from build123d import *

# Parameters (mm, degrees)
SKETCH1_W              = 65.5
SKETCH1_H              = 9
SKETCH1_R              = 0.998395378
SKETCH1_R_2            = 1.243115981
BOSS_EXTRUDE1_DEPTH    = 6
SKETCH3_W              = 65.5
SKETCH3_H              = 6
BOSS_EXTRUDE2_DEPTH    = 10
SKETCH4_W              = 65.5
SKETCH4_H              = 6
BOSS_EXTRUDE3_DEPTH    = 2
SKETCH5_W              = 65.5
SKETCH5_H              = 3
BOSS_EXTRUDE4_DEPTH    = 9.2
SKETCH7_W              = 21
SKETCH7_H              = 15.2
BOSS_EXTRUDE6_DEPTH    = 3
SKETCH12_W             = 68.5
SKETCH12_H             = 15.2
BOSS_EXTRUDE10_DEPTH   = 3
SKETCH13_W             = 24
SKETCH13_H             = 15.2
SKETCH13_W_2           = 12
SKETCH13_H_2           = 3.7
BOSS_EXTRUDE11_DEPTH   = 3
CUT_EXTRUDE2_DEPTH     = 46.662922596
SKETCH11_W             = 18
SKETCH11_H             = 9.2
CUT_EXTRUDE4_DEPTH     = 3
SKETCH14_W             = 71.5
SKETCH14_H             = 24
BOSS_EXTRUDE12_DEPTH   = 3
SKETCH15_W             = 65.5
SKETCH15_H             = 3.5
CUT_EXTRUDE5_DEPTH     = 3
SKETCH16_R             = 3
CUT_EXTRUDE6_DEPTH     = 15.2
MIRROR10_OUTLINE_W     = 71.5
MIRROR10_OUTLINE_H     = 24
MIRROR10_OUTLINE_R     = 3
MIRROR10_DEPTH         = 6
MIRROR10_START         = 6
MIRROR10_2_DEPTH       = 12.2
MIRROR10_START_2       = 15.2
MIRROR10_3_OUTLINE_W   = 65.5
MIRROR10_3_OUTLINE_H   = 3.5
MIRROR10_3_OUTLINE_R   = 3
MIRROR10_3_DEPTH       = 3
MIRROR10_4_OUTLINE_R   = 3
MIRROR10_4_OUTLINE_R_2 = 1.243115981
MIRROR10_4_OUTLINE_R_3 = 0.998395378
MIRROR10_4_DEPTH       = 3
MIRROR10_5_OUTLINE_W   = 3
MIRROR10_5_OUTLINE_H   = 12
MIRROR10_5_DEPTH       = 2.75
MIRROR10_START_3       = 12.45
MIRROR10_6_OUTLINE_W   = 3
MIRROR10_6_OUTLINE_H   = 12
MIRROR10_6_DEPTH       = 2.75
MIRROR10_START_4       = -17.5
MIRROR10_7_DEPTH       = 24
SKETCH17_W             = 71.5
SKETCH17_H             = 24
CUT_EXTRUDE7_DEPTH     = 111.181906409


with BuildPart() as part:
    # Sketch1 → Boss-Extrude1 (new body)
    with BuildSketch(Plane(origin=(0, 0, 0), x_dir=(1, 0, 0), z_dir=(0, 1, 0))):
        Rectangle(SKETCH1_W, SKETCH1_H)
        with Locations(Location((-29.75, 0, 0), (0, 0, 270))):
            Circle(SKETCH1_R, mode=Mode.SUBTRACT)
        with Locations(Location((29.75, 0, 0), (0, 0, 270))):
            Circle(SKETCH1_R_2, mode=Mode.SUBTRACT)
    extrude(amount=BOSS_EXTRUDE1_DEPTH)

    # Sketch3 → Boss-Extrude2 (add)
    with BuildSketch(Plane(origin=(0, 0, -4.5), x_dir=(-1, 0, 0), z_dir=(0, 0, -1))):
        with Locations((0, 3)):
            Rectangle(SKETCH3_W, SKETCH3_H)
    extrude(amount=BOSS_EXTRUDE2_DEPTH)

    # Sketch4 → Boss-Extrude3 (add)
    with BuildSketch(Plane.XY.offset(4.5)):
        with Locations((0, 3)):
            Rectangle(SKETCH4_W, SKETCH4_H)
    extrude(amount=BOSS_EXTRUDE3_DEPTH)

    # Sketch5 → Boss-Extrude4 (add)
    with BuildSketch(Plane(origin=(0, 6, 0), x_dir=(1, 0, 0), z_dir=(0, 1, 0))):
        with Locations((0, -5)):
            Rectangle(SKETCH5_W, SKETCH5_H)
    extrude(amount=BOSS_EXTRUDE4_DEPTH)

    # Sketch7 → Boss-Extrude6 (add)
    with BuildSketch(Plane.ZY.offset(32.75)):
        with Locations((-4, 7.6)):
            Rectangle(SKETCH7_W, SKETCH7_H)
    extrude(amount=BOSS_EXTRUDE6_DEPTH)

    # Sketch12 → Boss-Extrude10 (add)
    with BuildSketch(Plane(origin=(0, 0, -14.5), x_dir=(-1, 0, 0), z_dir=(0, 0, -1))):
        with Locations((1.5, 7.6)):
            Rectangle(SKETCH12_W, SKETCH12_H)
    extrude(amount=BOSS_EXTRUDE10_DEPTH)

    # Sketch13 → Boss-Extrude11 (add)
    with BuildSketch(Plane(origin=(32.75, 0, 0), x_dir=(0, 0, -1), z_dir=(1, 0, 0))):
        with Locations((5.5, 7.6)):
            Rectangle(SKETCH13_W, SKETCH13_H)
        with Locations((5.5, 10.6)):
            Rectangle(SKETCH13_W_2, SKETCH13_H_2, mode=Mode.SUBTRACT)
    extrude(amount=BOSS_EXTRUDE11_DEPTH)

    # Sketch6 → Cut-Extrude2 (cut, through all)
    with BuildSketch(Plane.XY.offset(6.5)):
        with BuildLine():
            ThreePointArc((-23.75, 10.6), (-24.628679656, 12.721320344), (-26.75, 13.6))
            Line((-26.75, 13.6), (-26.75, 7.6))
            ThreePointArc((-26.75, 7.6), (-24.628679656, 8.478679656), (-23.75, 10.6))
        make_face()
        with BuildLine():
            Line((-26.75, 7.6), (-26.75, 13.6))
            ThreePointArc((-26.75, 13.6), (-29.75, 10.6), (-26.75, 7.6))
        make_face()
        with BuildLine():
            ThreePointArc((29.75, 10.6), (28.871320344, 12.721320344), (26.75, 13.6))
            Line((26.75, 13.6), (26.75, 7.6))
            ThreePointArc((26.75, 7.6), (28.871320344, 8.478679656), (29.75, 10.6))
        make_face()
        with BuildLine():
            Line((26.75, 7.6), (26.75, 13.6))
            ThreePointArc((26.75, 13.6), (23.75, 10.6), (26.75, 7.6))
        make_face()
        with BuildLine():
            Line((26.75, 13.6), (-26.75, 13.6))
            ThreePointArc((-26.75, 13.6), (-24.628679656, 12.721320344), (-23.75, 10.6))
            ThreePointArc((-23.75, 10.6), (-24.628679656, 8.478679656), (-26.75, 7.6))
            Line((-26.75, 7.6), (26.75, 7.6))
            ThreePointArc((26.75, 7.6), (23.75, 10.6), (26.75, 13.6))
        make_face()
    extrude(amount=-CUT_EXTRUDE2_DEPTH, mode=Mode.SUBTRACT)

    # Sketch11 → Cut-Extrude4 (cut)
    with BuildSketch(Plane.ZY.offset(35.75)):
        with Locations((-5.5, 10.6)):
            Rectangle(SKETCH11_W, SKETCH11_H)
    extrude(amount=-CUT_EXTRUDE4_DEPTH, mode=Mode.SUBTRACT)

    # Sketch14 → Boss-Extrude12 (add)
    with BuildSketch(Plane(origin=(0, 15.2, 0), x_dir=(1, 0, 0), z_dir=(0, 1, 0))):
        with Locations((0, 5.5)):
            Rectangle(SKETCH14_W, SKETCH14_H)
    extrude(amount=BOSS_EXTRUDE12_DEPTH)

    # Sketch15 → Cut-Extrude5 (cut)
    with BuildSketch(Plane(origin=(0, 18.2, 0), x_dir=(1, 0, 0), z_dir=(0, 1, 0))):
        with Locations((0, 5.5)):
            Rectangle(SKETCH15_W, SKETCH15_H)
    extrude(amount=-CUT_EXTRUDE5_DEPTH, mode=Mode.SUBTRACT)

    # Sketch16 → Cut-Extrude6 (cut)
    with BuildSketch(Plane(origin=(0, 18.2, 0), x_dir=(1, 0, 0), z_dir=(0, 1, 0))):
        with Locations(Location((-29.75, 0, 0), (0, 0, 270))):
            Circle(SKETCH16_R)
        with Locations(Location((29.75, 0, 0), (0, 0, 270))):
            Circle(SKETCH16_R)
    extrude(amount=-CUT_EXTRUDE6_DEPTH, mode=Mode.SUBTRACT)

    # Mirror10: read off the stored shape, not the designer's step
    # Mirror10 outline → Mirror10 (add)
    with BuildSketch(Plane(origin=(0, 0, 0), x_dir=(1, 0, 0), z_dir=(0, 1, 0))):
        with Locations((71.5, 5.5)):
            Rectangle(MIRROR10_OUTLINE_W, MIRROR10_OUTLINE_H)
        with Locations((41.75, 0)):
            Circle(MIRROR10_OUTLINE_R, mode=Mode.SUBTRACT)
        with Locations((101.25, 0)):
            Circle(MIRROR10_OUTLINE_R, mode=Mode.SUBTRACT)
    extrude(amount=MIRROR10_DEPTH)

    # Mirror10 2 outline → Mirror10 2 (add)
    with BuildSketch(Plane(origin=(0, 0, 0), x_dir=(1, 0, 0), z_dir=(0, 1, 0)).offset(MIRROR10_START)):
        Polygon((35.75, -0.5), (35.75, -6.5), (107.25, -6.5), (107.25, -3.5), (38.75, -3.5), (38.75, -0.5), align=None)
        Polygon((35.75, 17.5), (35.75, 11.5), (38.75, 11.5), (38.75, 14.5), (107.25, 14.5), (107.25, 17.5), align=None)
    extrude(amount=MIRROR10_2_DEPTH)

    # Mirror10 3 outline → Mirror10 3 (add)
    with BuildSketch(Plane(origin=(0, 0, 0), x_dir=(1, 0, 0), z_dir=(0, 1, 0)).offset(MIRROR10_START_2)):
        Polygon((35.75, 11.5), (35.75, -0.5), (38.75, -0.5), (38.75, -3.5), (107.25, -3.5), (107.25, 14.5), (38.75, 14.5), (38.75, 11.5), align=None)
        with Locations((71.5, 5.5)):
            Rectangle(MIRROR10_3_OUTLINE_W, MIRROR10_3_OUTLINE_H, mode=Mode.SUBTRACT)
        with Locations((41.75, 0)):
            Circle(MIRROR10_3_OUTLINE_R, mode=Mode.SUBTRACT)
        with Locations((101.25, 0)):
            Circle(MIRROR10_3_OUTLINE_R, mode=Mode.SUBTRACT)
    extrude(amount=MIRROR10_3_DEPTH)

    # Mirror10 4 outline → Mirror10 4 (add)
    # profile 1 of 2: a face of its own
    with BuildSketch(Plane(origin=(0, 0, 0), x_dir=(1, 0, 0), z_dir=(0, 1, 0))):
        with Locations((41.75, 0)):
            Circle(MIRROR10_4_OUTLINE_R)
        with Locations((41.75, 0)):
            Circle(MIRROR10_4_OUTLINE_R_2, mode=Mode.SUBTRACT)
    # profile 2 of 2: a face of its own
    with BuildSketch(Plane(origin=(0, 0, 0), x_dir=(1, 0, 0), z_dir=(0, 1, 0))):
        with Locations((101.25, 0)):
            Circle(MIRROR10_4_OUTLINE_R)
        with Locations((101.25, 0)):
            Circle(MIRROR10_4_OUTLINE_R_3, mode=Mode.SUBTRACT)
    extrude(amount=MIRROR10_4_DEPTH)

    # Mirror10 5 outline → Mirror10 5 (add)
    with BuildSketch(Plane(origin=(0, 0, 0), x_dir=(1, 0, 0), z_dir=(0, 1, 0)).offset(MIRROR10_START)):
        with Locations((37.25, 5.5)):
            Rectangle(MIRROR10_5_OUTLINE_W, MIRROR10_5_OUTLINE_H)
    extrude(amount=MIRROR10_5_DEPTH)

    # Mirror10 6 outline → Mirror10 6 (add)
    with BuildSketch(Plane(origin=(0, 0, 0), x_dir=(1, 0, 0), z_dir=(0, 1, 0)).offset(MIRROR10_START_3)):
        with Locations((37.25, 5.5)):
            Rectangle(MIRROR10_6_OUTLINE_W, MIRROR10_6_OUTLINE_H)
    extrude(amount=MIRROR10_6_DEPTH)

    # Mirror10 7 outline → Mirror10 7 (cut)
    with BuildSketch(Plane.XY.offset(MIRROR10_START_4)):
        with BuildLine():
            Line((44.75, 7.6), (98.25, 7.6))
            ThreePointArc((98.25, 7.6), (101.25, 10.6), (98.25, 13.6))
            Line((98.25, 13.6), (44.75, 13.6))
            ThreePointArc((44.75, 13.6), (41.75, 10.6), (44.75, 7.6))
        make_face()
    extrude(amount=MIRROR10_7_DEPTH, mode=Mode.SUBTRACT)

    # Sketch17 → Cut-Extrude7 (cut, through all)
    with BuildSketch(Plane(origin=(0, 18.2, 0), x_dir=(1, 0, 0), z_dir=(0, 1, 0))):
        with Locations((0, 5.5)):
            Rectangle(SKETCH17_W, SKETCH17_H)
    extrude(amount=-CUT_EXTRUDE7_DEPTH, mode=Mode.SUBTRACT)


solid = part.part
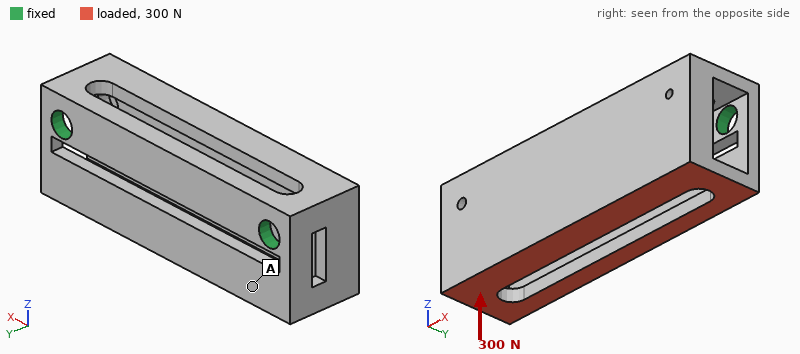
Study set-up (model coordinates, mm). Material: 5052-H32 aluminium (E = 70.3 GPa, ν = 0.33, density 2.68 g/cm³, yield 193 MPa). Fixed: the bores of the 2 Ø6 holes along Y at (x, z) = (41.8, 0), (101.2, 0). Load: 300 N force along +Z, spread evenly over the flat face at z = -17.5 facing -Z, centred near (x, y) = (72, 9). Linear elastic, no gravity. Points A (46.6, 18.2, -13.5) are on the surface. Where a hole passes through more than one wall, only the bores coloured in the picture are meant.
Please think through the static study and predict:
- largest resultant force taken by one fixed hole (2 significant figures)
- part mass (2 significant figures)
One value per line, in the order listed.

150 N
45 g
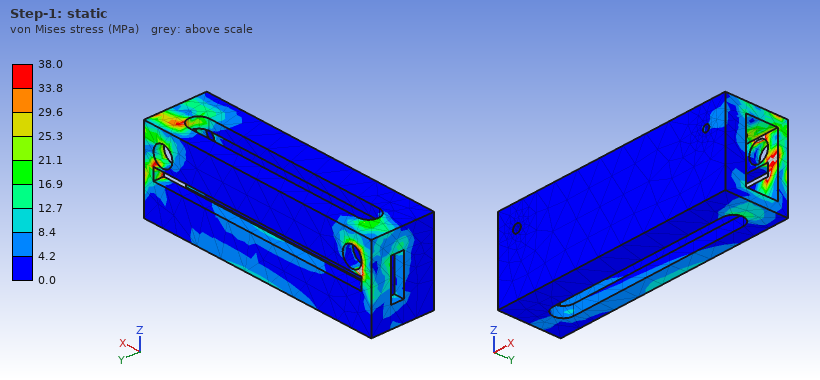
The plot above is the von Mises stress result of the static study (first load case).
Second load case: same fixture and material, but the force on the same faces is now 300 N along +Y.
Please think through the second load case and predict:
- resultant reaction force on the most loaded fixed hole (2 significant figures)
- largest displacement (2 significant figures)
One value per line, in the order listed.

160 N
0.10 mm
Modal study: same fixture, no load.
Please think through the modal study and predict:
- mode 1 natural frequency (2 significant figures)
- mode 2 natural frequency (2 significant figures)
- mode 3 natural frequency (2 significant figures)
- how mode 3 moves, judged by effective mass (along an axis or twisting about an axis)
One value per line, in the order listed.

2000 Hz
4100 Hz
4700 Hz
along X
